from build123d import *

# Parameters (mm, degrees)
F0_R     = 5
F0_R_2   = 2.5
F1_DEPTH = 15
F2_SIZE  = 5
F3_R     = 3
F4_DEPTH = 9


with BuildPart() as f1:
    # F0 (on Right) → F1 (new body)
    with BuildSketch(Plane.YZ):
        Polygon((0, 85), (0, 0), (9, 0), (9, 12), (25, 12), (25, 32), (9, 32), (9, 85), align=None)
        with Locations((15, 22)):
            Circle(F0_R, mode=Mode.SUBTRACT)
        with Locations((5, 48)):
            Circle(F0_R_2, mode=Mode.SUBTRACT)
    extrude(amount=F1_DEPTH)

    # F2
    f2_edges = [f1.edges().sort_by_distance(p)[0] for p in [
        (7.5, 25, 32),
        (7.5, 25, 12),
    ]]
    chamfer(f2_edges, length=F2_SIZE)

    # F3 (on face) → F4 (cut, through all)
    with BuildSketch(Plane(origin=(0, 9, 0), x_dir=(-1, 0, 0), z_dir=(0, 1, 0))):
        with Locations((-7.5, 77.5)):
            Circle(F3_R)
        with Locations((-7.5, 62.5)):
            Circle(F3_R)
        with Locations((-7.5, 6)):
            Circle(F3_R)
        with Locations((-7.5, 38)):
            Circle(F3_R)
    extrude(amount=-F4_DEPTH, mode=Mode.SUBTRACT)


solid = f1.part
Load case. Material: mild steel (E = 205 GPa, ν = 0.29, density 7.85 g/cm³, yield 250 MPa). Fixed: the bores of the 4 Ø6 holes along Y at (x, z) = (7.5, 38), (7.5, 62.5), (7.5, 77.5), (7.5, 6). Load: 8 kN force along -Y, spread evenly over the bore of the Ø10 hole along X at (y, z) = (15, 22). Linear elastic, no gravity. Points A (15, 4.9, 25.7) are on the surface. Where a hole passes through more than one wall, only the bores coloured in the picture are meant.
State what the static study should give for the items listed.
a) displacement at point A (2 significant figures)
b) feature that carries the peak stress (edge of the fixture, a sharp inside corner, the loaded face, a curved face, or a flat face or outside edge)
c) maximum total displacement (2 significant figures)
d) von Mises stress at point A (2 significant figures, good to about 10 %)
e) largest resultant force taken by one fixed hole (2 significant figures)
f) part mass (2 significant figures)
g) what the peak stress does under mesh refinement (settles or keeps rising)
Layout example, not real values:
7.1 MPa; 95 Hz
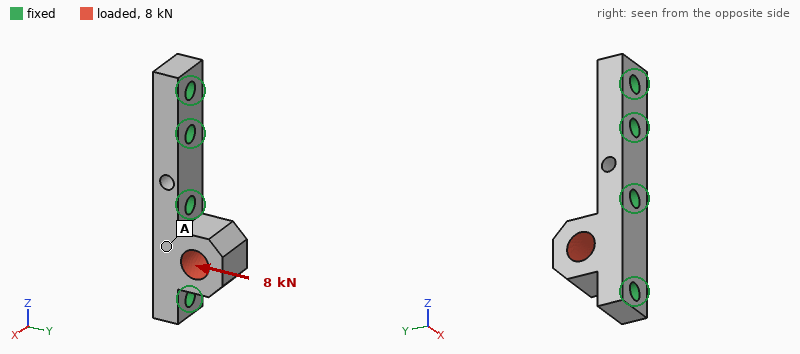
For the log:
5.1 µm; edge of the fixture; 6.6 µm; 15 MPa; 4.2 kN; 110 g; keeps rising
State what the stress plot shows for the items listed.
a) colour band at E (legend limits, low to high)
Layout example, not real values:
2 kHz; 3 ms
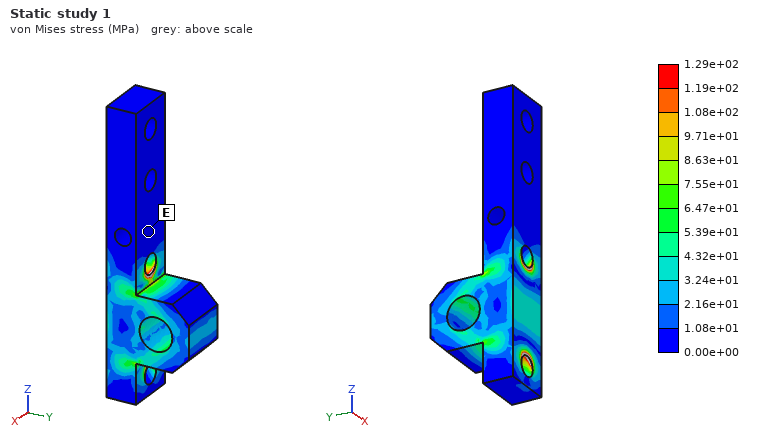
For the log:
0.00e+00 to 1.08e+01 MPa
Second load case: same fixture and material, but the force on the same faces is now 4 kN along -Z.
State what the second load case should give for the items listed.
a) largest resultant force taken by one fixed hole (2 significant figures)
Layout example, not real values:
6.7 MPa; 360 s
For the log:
2.5 kN
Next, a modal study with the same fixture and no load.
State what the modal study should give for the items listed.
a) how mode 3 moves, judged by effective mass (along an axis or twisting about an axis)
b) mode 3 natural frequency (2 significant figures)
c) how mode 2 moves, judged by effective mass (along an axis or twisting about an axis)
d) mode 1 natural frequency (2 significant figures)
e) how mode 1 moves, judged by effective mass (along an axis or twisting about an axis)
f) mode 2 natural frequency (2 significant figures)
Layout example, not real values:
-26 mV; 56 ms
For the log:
along Y; 30 kHz; along Z; 14 kHz; along X; 22 kHz
